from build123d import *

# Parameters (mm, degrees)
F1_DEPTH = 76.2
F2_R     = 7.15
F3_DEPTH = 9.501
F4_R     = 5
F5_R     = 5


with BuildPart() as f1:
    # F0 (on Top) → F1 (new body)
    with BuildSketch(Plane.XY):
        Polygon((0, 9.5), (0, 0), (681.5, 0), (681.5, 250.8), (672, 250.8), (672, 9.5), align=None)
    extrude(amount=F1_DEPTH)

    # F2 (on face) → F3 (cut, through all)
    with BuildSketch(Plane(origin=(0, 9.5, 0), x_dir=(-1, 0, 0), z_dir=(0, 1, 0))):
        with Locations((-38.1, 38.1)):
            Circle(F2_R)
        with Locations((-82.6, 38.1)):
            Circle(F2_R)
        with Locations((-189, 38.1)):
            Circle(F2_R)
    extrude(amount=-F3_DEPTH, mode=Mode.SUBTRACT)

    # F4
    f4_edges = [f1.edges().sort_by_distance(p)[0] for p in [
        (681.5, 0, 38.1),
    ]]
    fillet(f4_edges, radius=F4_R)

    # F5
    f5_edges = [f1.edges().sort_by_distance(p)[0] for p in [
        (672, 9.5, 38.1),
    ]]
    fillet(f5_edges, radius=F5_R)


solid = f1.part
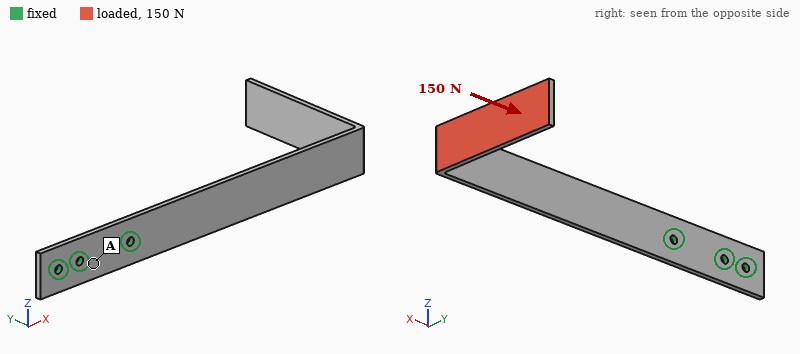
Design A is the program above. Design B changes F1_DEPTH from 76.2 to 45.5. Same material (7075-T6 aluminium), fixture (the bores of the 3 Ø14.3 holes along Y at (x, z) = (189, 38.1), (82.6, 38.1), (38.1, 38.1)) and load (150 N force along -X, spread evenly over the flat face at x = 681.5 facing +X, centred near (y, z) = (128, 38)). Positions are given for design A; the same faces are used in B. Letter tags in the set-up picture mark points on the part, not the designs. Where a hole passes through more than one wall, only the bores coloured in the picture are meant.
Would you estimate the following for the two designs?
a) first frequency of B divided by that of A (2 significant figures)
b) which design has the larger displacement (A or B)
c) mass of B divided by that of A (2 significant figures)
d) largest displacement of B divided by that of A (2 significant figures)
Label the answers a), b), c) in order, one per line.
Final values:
a) 1.00
b) B
c) 0.59
d) 1.7
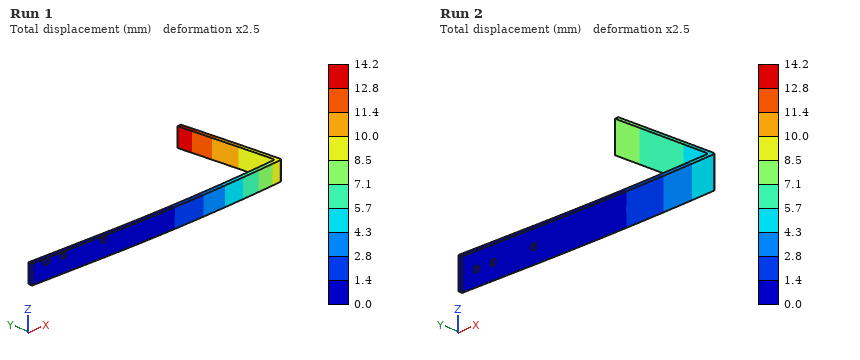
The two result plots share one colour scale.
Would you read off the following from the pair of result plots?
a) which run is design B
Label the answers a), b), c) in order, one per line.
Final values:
a) Run 1
